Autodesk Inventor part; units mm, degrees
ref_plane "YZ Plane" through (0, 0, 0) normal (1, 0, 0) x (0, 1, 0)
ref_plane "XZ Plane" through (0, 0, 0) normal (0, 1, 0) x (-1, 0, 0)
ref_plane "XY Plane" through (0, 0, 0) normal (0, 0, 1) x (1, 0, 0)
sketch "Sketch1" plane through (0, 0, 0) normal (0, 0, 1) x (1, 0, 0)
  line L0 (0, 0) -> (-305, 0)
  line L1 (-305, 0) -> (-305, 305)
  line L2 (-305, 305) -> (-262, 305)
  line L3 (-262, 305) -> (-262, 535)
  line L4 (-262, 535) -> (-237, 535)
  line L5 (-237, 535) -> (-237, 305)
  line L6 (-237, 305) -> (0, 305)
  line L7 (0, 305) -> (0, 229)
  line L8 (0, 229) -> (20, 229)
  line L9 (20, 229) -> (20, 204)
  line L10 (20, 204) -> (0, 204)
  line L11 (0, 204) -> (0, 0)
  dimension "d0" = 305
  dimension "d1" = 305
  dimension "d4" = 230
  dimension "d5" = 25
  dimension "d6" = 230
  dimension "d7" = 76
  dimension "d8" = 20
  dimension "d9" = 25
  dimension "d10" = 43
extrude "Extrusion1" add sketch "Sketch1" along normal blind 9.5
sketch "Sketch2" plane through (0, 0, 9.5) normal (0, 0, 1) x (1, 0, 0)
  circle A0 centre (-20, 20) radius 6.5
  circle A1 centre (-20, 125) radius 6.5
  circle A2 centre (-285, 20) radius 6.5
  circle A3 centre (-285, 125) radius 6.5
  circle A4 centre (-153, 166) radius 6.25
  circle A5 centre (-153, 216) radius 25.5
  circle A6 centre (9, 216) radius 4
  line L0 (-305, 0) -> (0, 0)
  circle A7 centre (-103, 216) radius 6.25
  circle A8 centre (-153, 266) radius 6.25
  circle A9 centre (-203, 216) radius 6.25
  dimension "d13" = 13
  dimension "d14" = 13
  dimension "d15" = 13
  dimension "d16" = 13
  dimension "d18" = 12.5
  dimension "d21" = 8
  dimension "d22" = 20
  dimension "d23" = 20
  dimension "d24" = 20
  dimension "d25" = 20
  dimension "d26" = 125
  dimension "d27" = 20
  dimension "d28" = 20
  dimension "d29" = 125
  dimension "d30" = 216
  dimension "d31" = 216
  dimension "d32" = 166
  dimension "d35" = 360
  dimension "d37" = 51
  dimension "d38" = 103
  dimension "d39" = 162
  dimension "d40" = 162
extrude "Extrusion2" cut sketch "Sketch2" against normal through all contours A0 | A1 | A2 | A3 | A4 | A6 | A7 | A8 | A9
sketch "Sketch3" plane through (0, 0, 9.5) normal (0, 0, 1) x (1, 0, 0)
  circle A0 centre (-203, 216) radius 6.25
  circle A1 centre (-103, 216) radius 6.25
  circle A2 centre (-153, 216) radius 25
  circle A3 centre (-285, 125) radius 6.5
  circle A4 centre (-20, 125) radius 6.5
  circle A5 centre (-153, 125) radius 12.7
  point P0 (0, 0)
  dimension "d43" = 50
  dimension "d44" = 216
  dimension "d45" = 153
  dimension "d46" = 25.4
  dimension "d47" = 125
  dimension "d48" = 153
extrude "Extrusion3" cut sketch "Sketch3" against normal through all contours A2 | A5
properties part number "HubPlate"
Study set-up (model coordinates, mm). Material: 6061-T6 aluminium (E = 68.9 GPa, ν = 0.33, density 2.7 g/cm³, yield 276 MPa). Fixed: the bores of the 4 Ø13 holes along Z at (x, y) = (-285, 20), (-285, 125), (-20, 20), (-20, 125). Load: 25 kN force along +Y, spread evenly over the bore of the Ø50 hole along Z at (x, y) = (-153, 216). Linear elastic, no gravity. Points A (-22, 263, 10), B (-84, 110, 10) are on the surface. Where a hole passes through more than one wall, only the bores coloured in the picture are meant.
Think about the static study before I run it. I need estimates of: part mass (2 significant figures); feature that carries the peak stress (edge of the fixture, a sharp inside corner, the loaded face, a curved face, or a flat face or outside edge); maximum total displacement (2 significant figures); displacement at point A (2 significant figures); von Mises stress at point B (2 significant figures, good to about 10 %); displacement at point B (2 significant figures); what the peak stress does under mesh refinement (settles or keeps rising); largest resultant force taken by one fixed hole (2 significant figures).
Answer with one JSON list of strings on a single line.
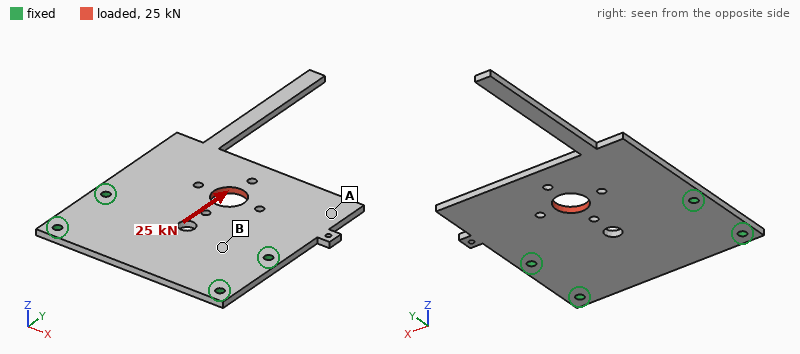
["2.5 kg", "edge of the fixture", "70 µm", "15 µm", "9.7 MPa", "18 µm", "keeps rising", "9.0 kN"]
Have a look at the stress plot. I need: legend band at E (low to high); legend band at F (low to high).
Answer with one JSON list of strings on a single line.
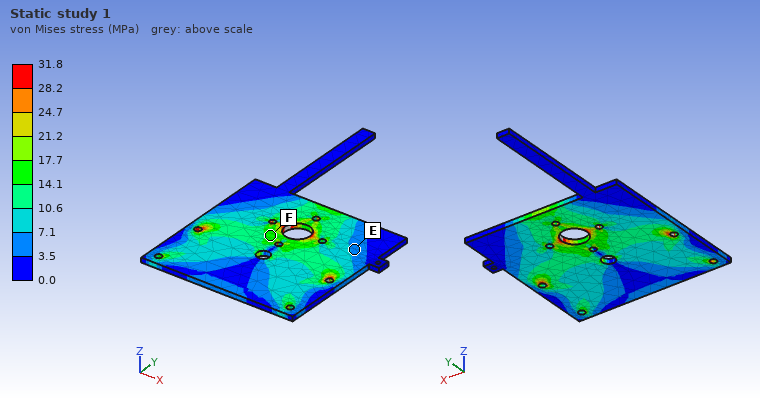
["3.5 to 7.1 MPa", "14.1 to 17.7 MPa"]
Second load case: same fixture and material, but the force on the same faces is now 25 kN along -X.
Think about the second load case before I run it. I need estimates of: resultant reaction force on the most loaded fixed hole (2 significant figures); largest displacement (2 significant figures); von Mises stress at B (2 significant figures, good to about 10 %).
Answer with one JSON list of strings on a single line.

["13 kN", "0.12 mm", "7.8 MPa"]
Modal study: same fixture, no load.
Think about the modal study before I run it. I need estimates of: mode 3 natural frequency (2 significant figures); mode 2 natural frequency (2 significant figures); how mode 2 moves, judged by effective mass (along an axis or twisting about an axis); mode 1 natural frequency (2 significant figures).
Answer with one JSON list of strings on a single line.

["350 Hz", "230 Hz", "along Z", "91 Hz"]
